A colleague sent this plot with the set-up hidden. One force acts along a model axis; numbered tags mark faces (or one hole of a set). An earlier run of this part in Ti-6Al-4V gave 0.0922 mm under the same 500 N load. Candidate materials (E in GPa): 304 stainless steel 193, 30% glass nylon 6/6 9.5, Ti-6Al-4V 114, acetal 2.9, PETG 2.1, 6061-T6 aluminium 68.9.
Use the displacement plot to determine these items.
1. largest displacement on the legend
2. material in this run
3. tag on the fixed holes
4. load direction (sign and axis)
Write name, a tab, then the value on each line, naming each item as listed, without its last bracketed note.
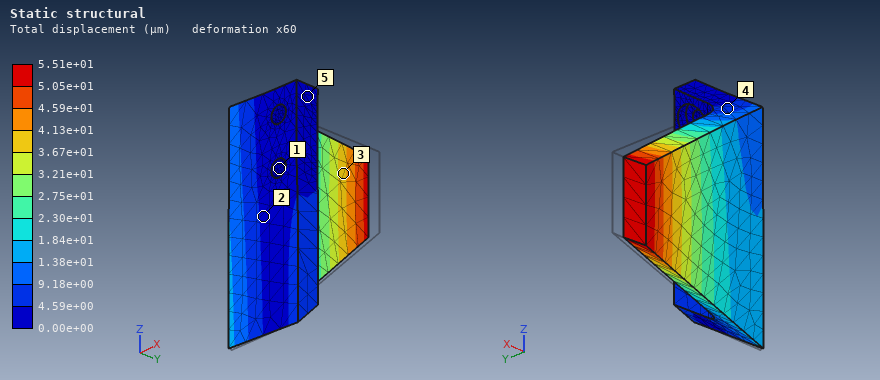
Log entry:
largest displacement on the legend	5.51e+01 µm
material in this run	304 stainless steel
tag on the fixed holes	1
load direction	-X
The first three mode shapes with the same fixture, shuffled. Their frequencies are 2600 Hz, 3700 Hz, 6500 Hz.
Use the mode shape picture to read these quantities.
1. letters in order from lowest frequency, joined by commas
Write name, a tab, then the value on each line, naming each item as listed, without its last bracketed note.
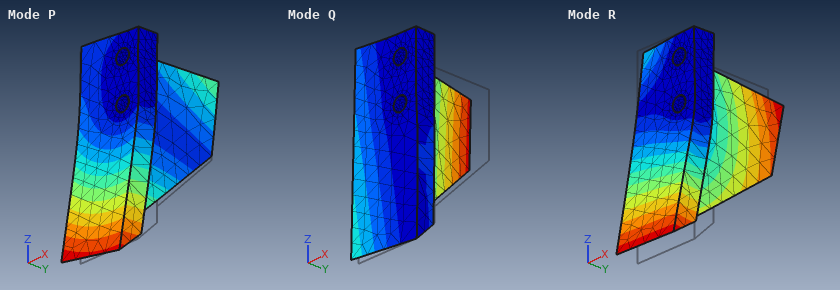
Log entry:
letters in order from lowest frequency, joined by commas	Q, R, P
